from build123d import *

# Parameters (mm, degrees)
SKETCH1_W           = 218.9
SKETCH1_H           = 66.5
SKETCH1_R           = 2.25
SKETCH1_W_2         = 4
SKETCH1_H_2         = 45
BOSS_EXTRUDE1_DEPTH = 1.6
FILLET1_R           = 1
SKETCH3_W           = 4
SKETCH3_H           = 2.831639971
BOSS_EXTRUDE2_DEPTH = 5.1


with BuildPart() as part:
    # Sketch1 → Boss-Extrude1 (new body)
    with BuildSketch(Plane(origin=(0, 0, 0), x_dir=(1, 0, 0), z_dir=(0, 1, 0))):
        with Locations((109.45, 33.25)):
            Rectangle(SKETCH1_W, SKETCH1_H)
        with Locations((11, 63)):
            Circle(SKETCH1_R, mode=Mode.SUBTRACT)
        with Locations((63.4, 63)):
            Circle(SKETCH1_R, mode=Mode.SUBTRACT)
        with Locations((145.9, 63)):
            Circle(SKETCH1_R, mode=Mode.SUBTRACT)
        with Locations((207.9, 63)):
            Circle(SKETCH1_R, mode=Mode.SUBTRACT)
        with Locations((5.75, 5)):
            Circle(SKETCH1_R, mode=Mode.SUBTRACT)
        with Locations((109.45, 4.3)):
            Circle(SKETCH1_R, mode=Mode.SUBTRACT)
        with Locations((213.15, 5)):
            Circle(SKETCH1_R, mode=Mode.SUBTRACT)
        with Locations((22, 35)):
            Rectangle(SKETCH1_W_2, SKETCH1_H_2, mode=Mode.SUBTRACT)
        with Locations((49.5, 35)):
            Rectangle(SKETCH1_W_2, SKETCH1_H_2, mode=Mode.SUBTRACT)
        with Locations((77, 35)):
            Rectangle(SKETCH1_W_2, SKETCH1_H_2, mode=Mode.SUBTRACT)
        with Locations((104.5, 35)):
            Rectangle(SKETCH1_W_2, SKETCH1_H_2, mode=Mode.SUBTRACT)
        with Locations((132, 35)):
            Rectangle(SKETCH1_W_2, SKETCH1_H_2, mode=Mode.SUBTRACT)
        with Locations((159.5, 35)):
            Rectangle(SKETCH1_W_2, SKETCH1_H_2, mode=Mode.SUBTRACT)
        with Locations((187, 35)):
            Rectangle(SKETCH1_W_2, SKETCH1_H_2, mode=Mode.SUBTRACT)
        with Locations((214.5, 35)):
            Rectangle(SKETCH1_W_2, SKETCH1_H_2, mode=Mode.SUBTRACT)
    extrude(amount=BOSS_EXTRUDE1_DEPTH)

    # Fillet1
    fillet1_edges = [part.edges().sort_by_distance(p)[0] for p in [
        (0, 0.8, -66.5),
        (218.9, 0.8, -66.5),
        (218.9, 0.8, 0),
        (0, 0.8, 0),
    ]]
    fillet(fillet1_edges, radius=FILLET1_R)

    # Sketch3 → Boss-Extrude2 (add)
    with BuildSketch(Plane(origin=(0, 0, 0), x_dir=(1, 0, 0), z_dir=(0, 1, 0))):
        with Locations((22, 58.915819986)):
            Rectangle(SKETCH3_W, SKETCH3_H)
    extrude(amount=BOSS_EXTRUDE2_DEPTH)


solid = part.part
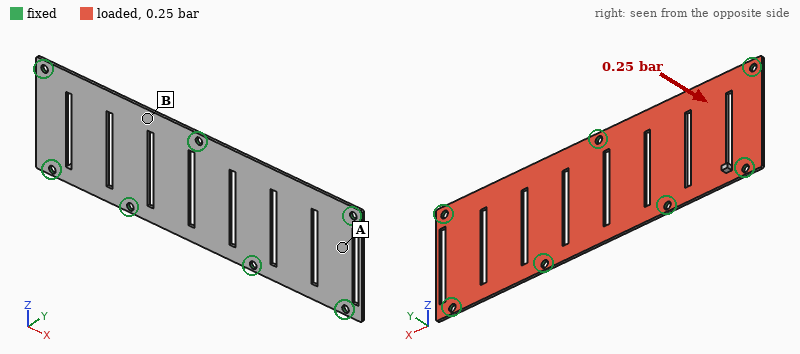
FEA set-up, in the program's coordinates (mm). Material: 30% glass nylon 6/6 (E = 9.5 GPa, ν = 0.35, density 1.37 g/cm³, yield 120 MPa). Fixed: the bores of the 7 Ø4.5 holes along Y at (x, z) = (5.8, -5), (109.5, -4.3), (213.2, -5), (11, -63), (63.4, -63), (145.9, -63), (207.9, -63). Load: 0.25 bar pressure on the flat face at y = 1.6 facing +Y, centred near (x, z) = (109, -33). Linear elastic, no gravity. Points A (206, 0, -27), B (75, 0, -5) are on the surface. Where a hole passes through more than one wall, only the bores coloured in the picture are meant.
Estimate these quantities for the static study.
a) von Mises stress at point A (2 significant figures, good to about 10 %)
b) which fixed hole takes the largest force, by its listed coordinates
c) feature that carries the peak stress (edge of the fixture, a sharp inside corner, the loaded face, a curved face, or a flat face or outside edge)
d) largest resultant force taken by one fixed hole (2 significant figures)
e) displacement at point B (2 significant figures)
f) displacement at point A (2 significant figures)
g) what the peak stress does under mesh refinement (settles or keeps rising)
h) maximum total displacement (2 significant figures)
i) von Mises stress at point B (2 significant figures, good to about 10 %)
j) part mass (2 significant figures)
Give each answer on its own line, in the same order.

11 MPa
(109.5, -4.3)
edge of the fixture
74 N
1.7 mm
0.40 mm
keeps rising
2.3 mm
22 MPa
29 g
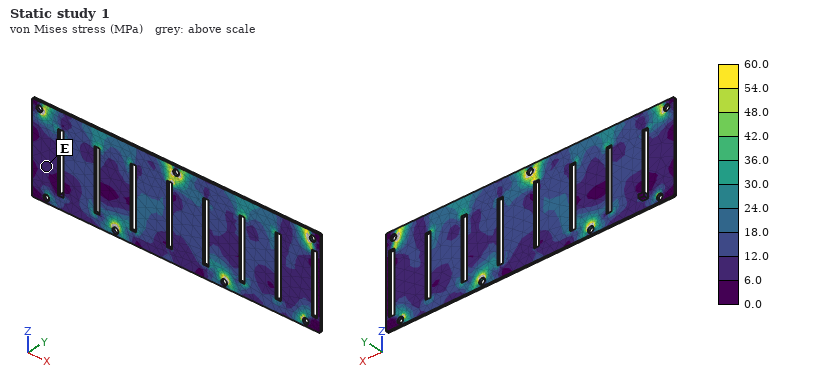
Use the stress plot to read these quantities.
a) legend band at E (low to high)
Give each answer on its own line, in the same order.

6.0 to 12.0 MPa
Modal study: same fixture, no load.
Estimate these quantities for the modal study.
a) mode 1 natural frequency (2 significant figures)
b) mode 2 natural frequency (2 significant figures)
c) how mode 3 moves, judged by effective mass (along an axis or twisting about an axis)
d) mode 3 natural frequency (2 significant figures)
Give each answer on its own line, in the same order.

430 Hz
450 Hz
along Y
610 Hz
